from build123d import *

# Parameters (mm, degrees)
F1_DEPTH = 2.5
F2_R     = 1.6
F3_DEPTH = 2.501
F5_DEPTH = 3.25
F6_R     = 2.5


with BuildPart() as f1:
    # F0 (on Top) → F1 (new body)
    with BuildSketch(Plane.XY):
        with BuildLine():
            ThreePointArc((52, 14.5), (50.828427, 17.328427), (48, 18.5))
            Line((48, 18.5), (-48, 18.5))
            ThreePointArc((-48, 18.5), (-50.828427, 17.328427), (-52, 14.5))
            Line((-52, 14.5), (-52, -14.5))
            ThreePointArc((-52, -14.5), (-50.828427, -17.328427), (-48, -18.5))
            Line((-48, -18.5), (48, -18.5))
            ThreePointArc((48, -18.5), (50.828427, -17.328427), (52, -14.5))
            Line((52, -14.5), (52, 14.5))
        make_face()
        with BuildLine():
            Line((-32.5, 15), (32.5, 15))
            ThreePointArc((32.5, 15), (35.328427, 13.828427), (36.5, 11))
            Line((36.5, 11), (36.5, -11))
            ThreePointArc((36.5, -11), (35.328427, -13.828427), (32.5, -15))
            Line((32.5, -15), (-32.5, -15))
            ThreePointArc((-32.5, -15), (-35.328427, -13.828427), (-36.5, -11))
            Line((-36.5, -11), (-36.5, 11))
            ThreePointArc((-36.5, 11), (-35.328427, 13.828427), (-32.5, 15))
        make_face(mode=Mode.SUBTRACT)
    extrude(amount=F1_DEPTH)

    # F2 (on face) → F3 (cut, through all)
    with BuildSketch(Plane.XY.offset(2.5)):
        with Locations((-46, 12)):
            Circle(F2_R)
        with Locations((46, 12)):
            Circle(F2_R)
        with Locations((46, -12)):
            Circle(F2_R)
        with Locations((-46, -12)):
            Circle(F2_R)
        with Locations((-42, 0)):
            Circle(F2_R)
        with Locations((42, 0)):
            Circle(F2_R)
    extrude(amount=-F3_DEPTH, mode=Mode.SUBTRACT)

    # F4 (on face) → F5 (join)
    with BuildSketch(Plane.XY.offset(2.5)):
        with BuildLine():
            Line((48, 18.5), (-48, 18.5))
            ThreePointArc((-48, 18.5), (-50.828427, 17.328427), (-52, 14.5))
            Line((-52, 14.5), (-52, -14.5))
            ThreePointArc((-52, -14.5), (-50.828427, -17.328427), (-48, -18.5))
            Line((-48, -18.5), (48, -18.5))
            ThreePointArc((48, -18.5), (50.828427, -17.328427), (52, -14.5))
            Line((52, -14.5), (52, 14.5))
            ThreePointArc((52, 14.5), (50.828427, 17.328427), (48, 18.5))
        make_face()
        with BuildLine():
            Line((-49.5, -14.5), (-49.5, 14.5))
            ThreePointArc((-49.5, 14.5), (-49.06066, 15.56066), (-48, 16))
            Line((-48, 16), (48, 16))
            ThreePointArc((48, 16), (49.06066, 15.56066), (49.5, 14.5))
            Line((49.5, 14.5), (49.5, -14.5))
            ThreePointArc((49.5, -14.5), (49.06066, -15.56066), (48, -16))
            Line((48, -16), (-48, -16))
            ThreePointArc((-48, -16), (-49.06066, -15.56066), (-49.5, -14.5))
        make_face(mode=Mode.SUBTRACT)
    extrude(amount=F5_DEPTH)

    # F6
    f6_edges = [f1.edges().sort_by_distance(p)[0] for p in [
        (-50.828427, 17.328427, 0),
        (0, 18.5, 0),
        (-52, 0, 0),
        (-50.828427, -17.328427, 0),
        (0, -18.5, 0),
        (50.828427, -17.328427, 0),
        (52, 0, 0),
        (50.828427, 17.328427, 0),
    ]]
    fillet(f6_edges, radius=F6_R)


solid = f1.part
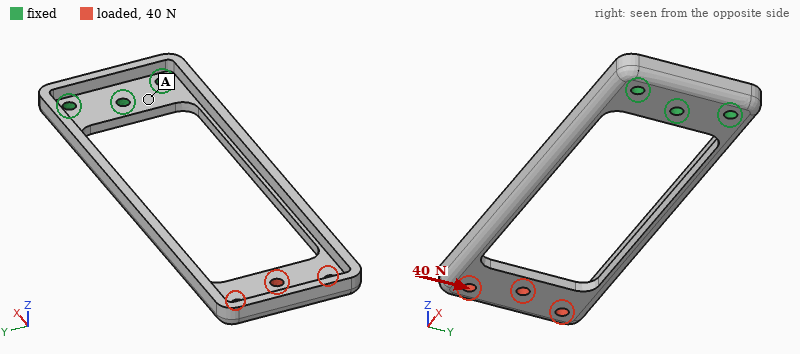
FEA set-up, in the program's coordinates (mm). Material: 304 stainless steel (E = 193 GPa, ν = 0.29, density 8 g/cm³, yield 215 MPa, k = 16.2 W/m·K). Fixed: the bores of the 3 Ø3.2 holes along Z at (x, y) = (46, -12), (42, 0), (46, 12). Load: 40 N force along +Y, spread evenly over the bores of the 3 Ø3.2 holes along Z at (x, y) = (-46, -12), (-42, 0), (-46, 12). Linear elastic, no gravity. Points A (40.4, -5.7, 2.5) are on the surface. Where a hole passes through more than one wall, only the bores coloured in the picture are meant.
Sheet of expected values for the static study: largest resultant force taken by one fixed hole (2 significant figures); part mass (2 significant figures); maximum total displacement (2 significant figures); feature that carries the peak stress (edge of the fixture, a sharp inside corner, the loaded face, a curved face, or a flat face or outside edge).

120 N
47 g
0.33 mm
a curved face
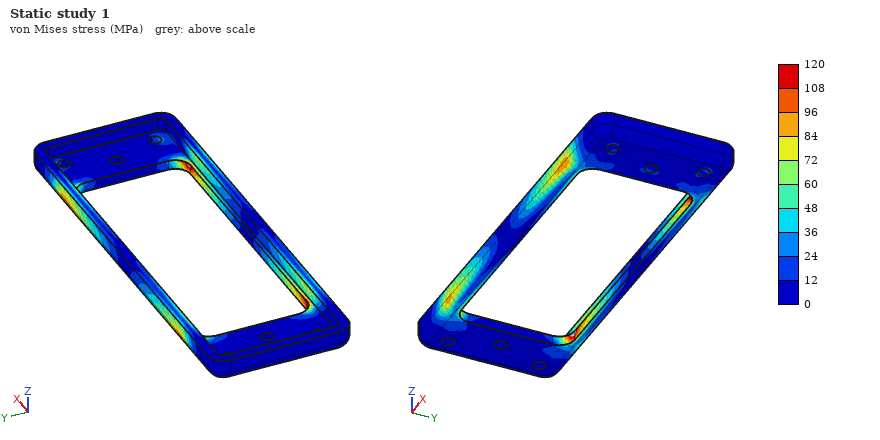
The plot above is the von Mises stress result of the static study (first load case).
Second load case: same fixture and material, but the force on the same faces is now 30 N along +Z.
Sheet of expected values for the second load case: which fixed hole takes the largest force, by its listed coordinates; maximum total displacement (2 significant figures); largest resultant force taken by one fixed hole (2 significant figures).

(42, 0)
0.55 mm
32 N
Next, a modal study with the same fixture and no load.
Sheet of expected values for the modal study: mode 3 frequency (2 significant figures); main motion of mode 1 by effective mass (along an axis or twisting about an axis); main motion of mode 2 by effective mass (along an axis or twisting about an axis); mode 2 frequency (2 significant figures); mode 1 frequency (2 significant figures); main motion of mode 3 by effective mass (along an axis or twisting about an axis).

820 Hz
along Z
along Y
390 Hz
290 Hz
twisting about X
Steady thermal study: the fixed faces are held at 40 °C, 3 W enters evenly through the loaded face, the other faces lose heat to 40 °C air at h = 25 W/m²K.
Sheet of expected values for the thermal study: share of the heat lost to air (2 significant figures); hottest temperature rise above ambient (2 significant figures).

98 %
59 K
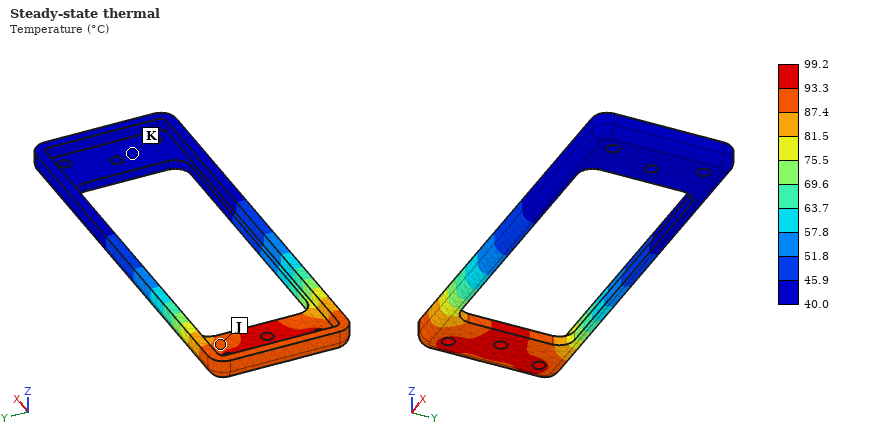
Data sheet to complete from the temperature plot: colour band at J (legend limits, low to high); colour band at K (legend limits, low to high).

87.4 to 93.3 °C
40.0 to 45.9 °C
